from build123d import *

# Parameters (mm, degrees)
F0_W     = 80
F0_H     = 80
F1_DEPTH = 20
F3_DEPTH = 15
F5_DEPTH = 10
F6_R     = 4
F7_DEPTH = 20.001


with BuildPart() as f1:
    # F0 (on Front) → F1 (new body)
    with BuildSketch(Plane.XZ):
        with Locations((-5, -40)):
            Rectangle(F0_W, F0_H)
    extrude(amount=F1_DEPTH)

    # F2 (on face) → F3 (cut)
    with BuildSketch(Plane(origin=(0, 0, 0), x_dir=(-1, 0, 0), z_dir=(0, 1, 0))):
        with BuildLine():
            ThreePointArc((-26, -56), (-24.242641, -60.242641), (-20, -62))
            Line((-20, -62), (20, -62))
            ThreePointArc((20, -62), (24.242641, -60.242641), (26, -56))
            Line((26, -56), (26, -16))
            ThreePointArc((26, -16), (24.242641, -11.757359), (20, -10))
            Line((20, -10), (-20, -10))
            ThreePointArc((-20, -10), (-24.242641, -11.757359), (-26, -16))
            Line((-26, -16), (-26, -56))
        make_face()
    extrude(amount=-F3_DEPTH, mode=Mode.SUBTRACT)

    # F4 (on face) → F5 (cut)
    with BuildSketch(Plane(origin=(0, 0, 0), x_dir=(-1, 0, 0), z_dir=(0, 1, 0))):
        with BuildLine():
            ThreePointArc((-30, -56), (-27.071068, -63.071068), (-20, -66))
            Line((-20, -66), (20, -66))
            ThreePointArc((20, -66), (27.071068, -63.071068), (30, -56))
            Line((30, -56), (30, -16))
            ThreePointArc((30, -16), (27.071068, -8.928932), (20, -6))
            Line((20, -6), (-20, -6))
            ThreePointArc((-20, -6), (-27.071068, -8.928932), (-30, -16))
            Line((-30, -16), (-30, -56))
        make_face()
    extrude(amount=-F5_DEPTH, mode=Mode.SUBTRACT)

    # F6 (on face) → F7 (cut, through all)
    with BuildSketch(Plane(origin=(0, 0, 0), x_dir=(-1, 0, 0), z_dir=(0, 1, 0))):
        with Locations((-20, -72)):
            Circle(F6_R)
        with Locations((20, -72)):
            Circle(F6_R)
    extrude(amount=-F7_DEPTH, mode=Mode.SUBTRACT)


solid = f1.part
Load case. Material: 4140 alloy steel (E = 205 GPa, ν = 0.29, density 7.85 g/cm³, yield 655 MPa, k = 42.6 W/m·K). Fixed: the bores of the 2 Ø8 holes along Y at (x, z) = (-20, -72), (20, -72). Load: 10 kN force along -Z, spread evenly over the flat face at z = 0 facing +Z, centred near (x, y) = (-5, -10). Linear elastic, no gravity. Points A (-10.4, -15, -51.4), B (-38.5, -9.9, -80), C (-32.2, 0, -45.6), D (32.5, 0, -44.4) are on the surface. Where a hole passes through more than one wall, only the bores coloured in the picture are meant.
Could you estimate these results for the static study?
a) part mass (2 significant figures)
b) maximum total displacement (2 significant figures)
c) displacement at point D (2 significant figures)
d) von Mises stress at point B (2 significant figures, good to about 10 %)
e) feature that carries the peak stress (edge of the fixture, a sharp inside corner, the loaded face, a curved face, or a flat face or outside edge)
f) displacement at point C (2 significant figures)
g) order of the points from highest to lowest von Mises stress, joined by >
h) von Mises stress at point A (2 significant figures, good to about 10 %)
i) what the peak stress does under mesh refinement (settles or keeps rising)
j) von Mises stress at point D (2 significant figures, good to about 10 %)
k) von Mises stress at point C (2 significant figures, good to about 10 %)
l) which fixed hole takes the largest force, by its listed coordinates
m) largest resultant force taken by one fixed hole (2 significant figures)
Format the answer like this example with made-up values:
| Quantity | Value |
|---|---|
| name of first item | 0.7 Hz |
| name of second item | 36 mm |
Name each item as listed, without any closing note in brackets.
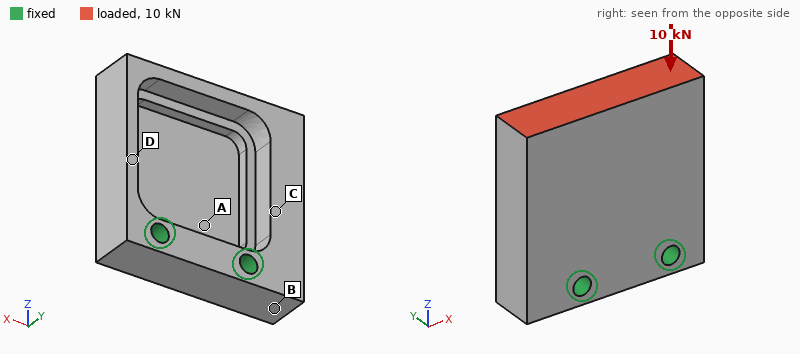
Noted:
| Quantity | Value |
|---|---|
| part mass | 610 g |
| maximum total displacement | 55 µm |
| displacement at point D | 9.2 µm |
| von Mises stress at point B | 10 MPa |
| feature that carries the peak stress | edge of the fixture |
| displacement at point C | 10 µm |
| order of the points from highest to lowest von Mises stress, joined by > | D > C > A > B |
| von Mises stress at point A | 24 MPa |
| what the peak stress does under mesh refinement | keeps rising |
| von Mises stress at point D | 51 MPa |
| von Mises stress at point C | 36 MPa |
| which fixed hole takes the largest force, by its listed coordinates | (-20, -72) |
| largest resultant force taken by one fixed hole | 5.9 kN |
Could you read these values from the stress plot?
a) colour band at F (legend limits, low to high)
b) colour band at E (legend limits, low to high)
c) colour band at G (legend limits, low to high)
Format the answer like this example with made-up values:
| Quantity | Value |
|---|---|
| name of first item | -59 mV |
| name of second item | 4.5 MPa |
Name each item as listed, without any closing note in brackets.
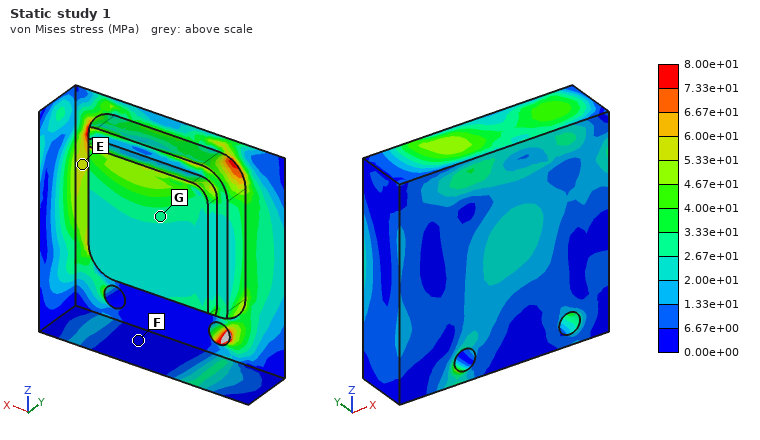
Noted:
| Quantity | Value |
|---|---|
| colour band at F | 0.00e+00 to 6.67e+00 MPa |
| colour band at E | 5.33e+01 to 6.00e+01 MPa |
| colour band at G | 2.67e+01 to 3.33e+01 MPa |
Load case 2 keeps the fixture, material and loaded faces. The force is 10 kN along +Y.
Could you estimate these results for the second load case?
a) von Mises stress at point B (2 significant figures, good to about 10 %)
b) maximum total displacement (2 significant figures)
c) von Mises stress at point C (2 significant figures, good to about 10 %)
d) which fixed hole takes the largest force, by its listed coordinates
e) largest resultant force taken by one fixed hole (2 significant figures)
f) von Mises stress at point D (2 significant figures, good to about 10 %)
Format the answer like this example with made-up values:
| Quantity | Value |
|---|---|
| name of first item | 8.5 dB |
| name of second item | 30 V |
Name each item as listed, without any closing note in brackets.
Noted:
| Quantity | Value |
|---|---|
| von Mises stress at point B | 130 MPa |
| maximum total displacement | 0.45 mm |
| von Mises stress at point C | 250 MPa |
| which fixed hole takes the largest force, by its listed coordinates | (-20, -72) |
| largest resultant force taken by one fixed hole | 6.5 kN |
| von Mises stress at point D | 380 MPa |
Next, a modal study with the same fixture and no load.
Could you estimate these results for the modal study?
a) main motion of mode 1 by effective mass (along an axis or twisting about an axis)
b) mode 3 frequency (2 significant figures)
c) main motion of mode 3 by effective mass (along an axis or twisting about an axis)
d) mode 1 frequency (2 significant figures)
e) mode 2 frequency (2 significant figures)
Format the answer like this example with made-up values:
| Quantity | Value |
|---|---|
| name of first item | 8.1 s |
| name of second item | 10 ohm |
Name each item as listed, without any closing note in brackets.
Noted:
| Quantity | Value |
|---|---|
| main motion of mode 1 by effective mass | along Y |
| mode 3 frequency | 5300 Hz |
| main motion of mode 3 by effective mass | along X |
| mode 1 frequency | 2000 Hz |
| mode 2 frequency | 3000 Hz |
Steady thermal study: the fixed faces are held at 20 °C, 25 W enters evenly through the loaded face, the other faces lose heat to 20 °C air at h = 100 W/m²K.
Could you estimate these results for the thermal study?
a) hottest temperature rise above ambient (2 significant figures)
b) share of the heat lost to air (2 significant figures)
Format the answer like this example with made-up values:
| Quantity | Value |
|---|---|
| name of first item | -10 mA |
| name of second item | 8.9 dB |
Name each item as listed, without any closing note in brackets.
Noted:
| Quantity | Value |
|---|---|
| hottest temperature rise above ambient | 29 K |
| share of the heat lost to air | 74 % |
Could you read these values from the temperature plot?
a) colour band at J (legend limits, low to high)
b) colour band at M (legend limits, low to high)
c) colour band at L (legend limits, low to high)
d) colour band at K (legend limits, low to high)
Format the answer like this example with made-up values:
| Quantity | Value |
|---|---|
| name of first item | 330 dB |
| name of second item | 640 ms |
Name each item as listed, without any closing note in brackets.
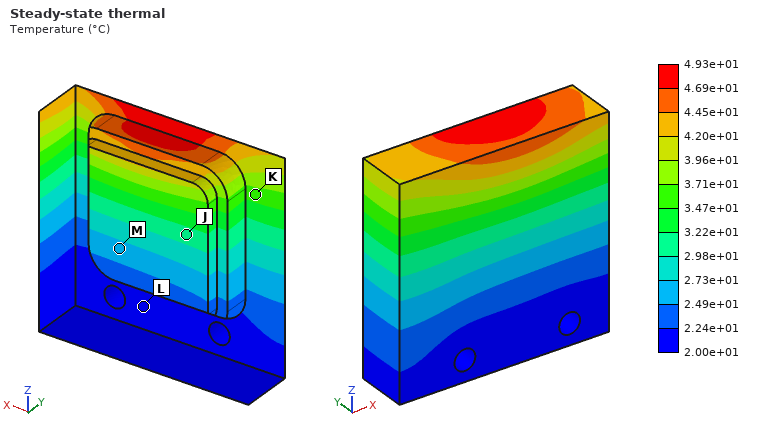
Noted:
| Quantity | Value |
|---|---|
| colour band at J | 2.98e+01 to 3.22e+01 °C |
| colour band at M | 2.49e+01 to 2.73e+01 °C |
| colour band at L | 2.00e+01 to 2.24e+01 °C |
| colour band at K | 3.47e+01 to 3.71e+01 °C |
